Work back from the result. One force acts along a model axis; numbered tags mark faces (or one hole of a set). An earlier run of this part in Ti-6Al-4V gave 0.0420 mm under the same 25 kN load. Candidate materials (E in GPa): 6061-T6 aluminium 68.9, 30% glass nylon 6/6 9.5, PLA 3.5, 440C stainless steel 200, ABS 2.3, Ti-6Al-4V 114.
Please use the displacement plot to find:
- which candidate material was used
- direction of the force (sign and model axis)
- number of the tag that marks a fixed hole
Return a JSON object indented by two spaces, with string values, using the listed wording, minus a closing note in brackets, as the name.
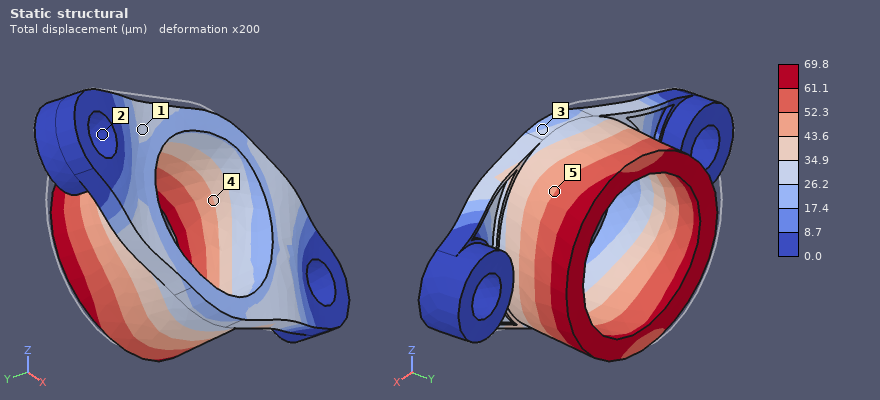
{
  "which candidate material was used": "6061-T6 aluminium",
  "direction of the force": "+X",
  "number of the tag that marks a fixed hole": "2"
}
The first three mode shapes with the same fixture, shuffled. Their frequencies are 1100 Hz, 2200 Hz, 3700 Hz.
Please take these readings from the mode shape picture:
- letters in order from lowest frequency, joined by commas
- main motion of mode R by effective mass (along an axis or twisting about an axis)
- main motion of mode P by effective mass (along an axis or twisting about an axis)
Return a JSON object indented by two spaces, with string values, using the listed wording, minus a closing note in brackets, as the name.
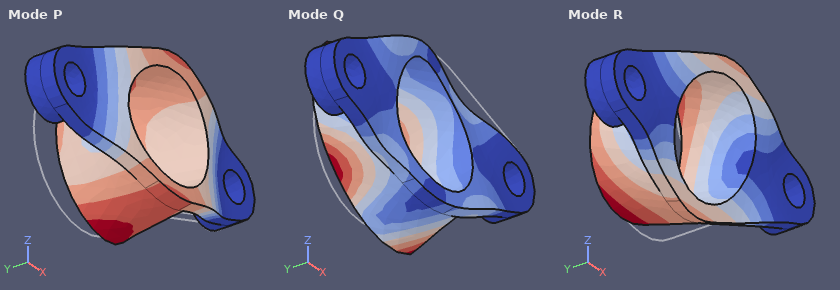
{
  "letters in order from lowest frequency, joined by commas": "R, P, Q",
  "main motion of mode R by effective mass": "along Z",
  "main motion of mode P by effective mass": "along Y"
}
